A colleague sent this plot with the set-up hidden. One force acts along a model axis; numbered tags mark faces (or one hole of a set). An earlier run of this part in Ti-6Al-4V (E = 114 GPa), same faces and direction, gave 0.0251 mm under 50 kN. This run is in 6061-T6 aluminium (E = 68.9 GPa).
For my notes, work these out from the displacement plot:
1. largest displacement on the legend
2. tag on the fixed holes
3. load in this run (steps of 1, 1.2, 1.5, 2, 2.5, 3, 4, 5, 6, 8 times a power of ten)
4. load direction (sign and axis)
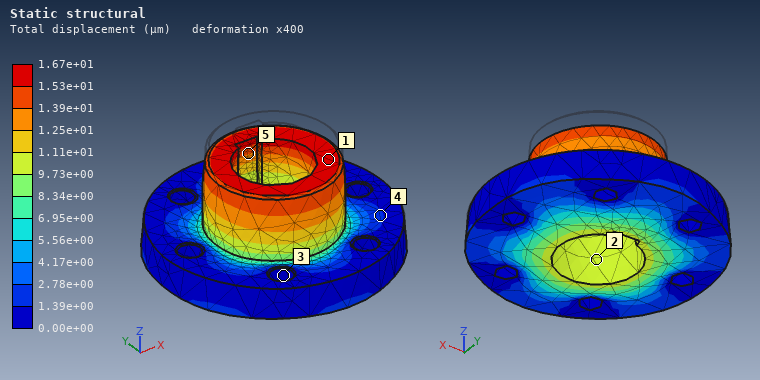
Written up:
1.67e+01 µm
3
20 kN
-Z
